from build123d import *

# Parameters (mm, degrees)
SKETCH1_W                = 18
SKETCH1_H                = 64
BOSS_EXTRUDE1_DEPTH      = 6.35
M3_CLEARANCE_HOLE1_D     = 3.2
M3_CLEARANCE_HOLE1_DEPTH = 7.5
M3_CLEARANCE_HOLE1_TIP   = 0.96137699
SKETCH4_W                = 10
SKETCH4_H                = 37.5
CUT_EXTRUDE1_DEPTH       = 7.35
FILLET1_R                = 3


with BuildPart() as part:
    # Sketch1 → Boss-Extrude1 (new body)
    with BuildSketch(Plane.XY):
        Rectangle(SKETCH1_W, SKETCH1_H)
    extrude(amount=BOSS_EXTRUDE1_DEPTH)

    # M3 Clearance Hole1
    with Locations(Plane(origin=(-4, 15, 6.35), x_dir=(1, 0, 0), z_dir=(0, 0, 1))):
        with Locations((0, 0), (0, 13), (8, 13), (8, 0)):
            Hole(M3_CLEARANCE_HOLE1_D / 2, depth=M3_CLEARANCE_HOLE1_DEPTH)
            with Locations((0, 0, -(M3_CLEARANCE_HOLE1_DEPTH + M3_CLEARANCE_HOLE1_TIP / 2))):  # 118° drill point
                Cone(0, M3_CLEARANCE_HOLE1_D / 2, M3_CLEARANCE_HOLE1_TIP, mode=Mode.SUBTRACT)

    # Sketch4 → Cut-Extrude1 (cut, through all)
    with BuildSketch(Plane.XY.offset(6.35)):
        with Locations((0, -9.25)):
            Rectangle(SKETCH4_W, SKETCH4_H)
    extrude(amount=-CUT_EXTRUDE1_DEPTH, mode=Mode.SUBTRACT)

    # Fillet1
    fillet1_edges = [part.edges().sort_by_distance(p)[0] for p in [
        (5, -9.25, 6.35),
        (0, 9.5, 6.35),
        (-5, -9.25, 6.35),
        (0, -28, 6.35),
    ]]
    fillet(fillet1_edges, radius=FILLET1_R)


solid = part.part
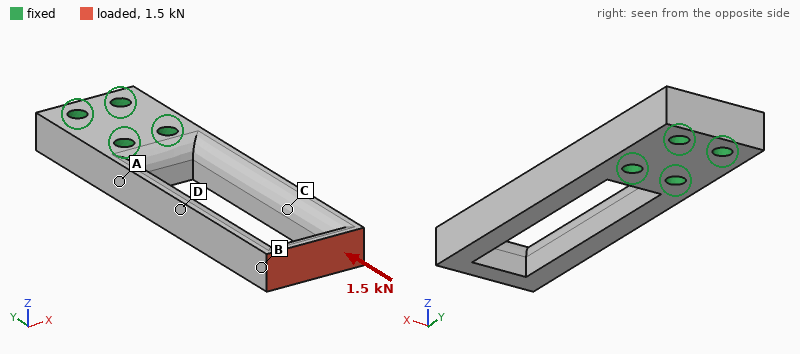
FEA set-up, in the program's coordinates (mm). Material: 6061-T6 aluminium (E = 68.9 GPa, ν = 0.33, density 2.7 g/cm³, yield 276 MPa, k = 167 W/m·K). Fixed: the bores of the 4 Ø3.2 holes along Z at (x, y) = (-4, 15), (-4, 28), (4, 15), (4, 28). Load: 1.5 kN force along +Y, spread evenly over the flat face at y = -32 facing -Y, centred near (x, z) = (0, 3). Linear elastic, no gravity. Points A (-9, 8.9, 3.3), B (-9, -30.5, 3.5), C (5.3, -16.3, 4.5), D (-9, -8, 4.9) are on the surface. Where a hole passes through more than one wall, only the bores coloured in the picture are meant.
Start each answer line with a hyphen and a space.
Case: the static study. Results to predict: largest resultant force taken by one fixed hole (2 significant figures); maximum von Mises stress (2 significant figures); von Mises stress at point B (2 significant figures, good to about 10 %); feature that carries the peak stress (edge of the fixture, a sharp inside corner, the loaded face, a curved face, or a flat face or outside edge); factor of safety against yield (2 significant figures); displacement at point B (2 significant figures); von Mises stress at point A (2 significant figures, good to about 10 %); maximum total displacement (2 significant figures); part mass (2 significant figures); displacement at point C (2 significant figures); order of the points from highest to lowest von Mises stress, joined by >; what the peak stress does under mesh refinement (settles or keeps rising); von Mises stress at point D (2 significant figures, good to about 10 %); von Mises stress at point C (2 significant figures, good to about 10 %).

- 650 N
- 100 MPa
- 12 MPa
- a curved face
- 2.7
- 35 µm
- 43 MPa
- 58 µm
- 12 g
- 31 µm
- C > A > D > B
- settles
- 26 MPa
- 57 MPa
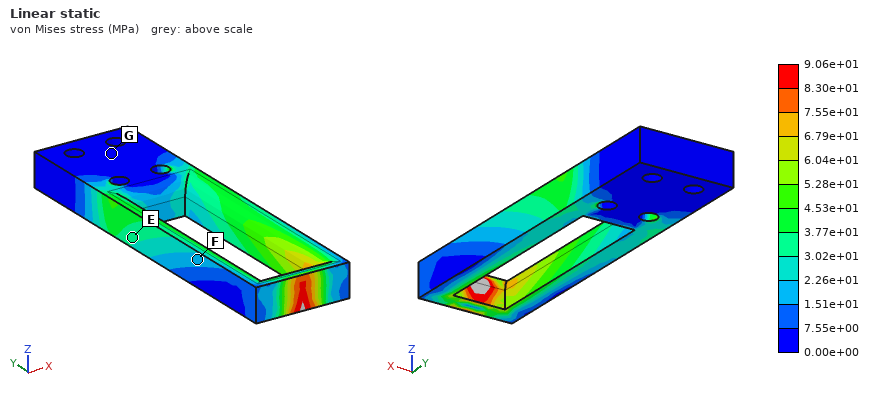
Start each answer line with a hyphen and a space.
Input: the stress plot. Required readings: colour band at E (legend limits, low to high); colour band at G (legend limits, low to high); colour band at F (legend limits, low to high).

- 3.02e+01 to 3.77e+01 MPa
- 0.00e+00 to 7.55e+00 MPa
- 1.51e+01 to 2.26e+01 MPa
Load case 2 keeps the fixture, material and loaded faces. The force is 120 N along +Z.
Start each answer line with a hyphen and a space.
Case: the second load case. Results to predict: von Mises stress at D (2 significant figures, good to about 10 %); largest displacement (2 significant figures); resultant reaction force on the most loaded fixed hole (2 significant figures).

- 39 MPa
- 0.39 mm
- 97 N
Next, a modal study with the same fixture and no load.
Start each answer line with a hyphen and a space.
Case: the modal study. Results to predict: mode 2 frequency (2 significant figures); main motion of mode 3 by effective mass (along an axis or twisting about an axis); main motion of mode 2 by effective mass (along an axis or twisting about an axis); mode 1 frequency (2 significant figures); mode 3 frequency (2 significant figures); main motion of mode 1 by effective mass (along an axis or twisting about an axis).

- 2200 Hz
- twisting about Y
- along X
- 2000 Hz
- 5300 Hz
- along Z
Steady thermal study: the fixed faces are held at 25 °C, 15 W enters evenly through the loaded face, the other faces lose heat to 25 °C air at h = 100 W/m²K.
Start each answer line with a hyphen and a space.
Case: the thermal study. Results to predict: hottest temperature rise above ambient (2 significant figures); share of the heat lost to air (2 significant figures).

- 63 K
- 38 %
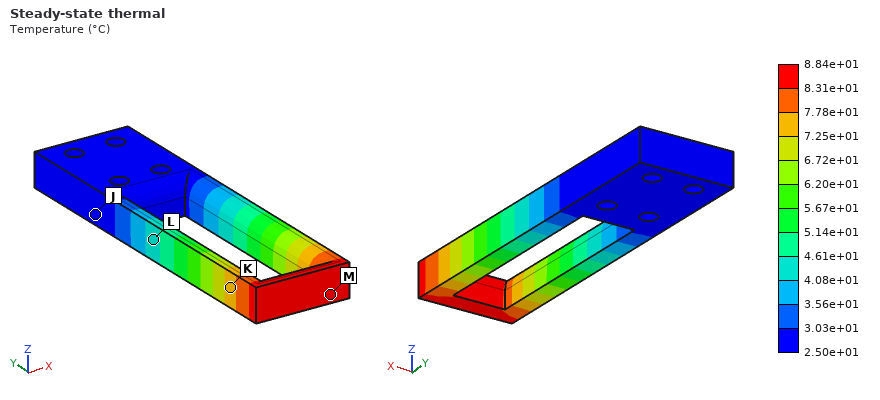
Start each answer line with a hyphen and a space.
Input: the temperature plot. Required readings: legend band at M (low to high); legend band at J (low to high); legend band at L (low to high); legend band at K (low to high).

- 8.31e+01 to 8.84e+01 °C
- 2.50e+01 to 3.03e+01 °C
- 4.08e+01 to 4.61e+01 °C
- 7.25e+01 to 7.78e+01 °C
